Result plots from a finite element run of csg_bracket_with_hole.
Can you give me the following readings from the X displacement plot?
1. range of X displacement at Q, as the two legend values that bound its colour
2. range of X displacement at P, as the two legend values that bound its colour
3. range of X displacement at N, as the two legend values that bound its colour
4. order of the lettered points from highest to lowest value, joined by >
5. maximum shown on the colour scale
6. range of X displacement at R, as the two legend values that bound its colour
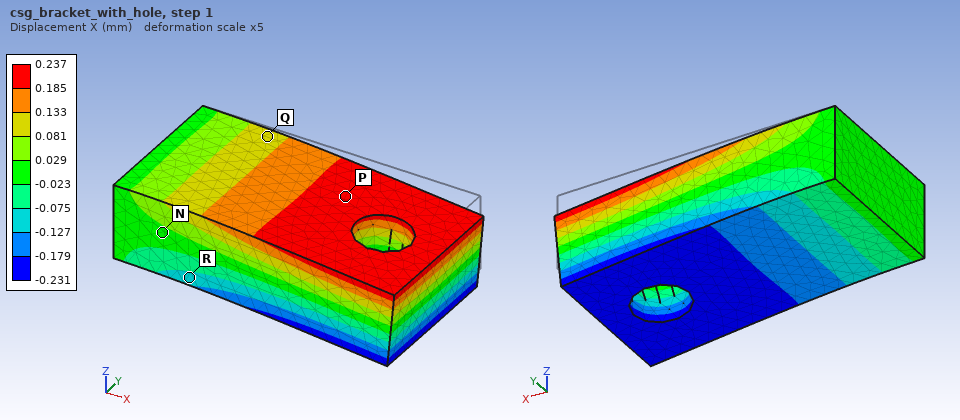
0.081 to 0.133 mm
0.185 to 0.237 mm
-0.023 to 0.029 mm
P > Q > N > R
0.237 mm
-0.127 to -0.075 mm
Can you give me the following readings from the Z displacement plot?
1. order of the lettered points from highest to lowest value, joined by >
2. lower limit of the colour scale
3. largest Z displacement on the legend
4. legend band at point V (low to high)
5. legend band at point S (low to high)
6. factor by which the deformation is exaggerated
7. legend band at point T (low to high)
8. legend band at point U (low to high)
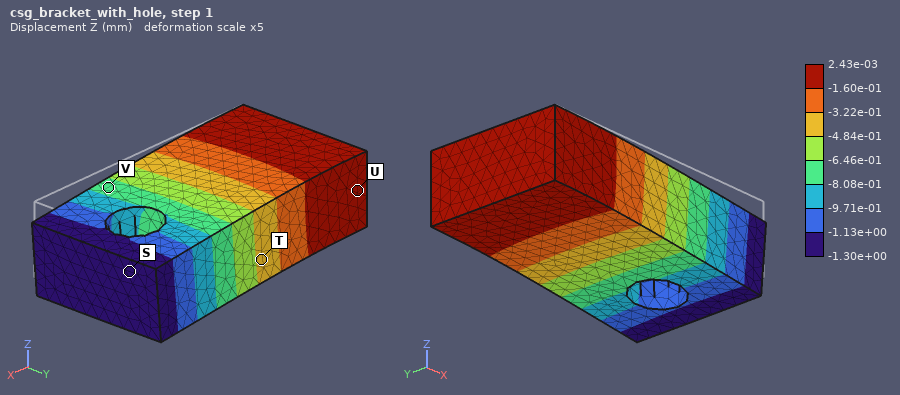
U > T > V > S
-1.30e+00 mm
2.43e-03 mm
-8.08e-01 to -6.46e-01 mm
-1.30e+00 to -1.13e+00 mm
5
-4.84e-01 to -3.22e-01 mm
-1.60e-01 to 2.43e-03 mm
